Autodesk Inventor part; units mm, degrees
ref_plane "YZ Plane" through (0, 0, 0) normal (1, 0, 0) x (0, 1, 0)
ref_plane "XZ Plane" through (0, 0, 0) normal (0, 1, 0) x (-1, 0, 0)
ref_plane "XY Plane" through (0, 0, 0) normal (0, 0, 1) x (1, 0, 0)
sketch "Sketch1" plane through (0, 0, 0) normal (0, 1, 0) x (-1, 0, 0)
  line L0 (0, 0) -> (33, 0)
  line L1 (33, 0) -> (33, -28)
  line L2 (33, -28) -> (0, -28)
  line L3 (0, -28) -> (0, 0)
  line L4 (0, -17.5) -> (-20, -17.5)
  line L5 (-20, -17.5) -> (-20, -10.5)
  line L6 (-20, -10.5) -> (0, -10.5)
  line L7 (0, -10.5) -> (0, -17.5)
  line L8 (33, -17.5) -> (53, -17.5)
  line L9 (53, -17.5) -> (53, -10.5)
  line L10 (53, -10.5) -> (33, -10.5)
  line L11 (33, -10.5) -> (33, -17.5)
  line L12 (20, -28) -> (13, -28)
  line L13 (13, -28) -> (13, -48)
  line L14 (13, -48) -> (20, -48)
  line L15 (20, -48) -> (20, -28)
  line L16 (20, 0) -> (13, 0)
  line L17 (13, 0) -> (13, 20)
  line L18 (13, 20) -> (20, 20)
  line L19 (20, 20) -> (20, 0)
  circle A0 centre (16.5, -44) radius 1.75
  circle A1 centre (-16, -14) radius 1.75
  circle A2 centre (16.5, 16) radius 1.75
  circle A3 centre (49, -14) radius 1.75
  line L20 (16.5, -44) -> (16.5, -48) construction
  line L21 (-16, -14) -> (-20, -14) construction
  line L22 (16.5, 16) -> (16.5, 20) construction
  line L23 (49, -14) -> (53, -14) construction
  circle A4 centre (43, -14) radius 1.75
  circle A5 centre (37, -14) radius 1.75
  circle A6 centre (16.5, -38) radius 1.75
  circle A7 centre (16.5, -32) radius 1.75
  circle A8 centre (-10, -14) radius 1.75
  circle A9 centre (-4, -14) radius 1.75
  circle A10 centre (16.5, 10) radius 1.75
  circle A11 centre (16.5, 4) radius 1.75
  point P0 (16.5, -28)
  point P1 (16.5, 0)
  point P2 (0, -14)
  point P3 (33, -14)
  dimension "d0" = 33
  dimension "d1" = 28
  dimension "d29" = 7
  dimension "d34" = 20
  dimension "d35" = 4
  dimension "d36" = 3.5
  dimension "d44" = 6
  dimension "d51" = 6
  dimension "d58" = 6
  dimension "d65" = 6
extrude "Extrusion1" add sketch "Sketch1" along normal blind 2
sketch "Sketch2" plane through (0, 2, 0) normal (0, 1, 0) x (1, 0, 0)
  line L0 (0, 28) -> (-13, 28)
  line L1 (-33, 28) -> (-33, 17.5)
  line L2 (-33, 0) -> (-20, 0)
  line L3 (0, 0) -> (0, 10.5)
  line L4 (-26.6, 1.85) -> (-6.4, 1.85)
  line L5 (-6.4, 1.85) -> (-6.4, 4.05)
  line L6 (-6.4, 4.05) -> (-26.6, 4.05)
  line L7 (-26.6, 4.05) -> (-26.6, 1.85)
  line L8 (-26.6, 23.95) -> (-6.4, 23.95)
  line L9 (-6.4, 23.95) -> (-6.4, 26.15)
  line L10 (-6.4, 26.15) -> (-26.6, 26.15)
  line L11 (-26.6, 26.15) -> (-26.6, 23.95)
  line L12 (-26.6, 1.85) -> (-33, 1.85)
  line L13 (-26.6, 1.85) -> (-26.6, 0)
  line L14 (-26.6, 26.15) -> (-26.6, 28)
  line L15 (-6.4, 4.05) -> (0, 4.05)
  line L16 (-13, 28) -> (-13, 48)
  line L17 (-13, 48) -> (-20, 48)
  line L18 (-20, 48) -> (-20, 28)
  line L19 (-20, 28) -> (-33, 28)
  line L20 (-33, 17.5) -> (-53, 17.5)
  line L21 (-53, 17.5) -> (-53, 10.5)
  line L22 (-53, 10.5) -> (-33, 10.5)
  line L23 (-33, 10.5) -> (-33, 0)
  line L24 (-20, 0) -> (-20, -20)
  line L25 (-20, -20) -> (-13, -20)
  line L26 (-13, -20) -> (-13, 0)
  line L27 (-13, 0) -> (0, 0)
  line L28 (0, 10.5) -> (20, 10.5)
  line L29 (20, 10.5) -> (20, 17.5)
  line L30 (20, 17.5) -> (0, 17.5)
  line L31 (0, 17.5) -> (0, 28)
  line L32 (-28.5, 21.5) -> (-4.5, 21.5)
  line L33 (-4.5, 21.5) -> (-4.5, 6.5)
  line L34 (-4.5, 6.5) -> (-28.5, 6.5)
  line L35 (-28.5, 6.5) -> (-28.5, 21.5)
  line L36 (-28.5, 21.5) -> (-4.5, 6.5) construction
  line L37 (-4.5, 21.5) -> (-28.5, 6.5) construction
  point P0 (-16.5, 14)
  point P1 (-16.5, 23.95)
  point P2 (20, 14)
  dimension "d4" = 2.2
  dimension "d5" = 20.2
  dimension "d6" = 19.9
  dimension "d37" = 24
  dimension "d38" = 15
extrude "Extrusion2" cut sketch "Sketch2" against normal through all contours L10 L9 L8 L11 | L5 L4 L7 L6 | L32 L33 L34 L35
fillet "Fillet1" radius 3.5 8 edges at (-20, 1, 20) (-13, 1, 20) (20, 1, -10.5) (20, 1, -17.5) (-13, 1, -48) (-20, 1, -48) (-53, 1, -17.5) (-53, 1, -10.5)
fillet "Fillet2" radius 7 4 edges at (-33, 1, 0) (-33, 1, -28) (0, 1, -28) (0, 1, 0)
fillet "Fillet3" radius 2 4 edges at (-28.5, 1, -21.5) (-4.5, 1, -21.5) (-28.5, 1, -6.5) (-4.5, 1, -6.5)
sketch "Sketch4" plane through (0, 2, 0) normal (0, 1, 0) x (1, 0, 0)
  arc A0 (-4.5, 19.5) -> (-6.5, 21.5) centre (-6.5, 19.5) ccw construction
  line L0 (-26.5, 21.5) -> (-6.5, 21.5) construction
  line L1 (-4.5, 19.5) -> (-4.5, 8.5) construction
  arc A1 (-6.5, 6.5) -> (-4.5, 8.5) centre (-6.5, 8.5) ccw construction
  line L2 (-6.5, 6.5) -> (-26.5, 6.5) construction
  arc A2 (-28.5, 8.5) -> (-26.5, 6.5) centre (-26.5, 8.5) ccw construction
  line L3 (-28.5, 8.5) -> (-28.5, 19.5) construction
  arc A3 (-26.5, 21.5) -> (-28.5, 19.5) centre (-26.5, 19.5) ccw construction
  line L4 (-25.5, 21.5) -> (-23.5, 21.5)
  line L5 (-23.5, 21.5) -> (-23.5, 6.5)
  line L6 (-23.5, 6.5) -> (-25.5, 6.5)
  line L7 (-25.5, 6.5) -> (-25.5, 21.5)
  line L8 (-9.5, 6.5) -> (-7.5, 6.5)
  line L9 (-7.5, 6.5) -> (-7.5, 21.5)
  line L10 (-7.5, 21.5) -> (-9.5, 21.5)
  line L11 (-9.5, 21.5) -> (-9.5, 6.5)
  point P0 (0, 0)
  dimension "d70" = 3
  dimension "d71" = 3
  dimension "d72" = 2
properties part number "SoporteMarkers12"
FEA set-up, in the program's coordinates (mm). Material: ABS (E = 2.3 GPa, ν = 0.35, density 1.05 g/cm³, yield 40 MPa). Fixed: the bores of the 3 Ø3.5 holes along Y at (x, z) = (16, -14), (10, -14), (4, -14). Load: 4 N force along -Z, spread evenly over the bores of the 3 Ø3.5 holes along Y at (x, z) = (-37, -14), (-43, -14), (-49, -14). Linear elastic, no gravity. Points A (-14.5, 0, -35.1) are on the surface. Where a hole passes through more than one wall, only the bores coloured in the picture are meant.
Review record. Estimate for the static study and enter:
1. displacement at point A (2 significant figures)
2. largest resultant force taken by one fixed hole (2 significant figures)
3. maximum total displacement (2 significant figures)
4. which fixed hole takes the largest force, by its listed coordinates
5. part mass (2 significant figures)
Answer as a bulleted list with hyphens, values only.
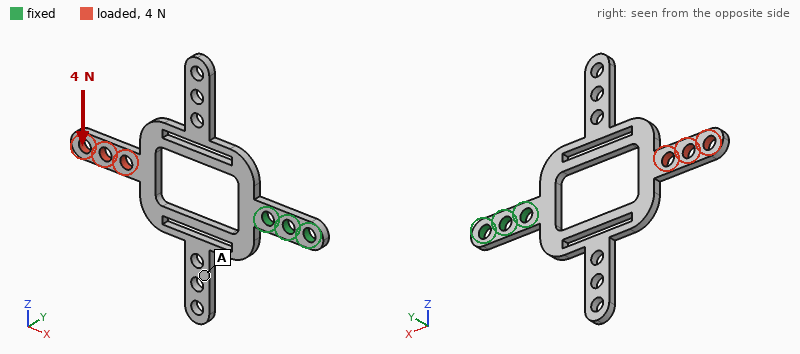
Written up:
- 0.57 mm
- 9.7 N
- 1.1 mm
- (4, -14)
- 1.8 g
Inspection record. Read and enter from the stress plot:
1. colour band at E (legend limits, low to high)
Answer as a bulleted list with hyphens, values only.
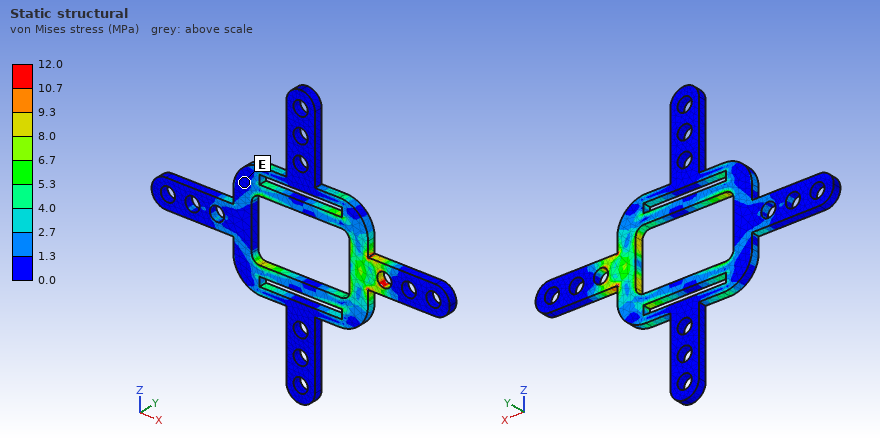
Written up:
- 0.0 to 1.3 MPa
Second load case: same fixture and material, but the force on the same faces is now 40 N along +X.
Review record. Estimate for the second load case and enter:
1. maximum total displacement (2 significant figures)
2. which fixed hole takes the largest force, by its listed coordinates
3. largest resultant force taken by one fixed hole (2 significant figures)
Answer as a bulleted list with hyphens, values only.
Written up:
- 0.20 mm
- (4, -14)
- 38 N
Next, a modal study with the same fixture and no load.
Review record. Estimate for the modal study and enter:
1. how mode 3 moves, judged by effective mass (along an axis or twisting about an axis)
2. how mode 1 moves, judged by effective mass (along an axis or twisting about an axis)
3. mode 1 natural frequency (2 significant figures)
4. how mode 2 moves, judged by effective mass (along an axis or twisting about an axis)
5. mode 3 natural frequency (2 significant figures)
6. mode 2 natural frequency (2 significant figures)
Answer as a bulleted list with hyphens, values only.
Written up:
- along Z
- along Y
- 150 Hz
- twisting about X
- 370 Hz
- 250 Hz
